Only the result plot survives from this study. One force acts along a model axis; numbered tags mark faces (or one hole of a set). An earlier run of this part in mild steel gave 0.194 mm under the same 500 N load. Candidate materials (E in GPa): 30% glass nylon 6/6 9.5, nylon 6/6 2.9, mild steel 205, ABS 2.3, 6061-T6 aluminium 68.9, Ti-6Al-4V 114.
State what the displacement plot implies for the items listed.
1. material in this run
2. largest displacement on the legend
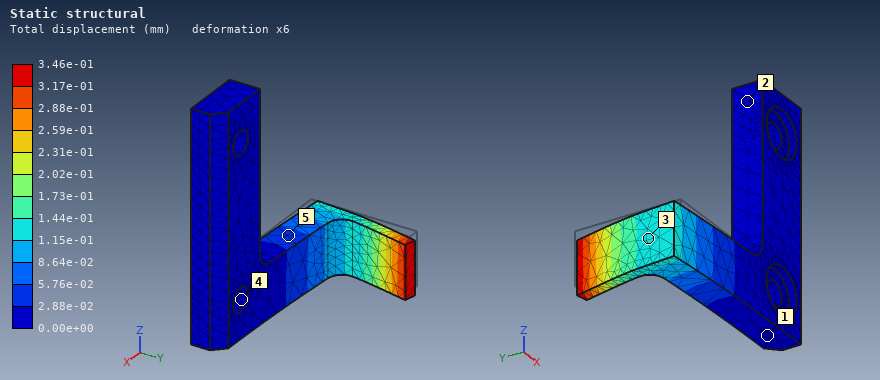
Ti-6Al-4V
3.46e-01 mm
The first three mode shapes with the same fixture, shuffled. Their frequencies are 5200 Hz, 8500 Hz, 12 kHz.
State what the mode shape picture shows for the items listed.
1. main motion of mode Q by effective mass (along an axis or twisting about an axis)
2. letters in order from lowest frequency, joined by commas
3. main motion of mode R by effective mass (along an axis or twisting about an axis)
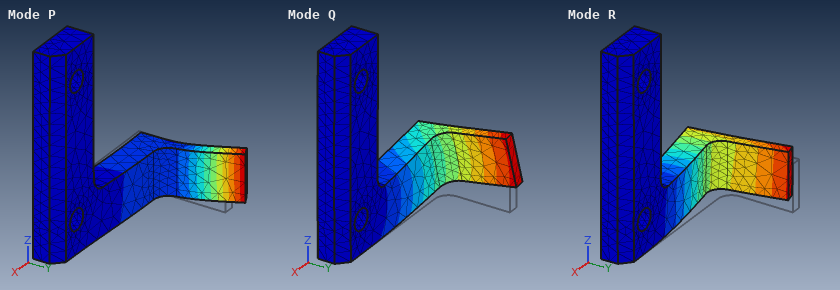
along Z
R, Q, P
along Y
